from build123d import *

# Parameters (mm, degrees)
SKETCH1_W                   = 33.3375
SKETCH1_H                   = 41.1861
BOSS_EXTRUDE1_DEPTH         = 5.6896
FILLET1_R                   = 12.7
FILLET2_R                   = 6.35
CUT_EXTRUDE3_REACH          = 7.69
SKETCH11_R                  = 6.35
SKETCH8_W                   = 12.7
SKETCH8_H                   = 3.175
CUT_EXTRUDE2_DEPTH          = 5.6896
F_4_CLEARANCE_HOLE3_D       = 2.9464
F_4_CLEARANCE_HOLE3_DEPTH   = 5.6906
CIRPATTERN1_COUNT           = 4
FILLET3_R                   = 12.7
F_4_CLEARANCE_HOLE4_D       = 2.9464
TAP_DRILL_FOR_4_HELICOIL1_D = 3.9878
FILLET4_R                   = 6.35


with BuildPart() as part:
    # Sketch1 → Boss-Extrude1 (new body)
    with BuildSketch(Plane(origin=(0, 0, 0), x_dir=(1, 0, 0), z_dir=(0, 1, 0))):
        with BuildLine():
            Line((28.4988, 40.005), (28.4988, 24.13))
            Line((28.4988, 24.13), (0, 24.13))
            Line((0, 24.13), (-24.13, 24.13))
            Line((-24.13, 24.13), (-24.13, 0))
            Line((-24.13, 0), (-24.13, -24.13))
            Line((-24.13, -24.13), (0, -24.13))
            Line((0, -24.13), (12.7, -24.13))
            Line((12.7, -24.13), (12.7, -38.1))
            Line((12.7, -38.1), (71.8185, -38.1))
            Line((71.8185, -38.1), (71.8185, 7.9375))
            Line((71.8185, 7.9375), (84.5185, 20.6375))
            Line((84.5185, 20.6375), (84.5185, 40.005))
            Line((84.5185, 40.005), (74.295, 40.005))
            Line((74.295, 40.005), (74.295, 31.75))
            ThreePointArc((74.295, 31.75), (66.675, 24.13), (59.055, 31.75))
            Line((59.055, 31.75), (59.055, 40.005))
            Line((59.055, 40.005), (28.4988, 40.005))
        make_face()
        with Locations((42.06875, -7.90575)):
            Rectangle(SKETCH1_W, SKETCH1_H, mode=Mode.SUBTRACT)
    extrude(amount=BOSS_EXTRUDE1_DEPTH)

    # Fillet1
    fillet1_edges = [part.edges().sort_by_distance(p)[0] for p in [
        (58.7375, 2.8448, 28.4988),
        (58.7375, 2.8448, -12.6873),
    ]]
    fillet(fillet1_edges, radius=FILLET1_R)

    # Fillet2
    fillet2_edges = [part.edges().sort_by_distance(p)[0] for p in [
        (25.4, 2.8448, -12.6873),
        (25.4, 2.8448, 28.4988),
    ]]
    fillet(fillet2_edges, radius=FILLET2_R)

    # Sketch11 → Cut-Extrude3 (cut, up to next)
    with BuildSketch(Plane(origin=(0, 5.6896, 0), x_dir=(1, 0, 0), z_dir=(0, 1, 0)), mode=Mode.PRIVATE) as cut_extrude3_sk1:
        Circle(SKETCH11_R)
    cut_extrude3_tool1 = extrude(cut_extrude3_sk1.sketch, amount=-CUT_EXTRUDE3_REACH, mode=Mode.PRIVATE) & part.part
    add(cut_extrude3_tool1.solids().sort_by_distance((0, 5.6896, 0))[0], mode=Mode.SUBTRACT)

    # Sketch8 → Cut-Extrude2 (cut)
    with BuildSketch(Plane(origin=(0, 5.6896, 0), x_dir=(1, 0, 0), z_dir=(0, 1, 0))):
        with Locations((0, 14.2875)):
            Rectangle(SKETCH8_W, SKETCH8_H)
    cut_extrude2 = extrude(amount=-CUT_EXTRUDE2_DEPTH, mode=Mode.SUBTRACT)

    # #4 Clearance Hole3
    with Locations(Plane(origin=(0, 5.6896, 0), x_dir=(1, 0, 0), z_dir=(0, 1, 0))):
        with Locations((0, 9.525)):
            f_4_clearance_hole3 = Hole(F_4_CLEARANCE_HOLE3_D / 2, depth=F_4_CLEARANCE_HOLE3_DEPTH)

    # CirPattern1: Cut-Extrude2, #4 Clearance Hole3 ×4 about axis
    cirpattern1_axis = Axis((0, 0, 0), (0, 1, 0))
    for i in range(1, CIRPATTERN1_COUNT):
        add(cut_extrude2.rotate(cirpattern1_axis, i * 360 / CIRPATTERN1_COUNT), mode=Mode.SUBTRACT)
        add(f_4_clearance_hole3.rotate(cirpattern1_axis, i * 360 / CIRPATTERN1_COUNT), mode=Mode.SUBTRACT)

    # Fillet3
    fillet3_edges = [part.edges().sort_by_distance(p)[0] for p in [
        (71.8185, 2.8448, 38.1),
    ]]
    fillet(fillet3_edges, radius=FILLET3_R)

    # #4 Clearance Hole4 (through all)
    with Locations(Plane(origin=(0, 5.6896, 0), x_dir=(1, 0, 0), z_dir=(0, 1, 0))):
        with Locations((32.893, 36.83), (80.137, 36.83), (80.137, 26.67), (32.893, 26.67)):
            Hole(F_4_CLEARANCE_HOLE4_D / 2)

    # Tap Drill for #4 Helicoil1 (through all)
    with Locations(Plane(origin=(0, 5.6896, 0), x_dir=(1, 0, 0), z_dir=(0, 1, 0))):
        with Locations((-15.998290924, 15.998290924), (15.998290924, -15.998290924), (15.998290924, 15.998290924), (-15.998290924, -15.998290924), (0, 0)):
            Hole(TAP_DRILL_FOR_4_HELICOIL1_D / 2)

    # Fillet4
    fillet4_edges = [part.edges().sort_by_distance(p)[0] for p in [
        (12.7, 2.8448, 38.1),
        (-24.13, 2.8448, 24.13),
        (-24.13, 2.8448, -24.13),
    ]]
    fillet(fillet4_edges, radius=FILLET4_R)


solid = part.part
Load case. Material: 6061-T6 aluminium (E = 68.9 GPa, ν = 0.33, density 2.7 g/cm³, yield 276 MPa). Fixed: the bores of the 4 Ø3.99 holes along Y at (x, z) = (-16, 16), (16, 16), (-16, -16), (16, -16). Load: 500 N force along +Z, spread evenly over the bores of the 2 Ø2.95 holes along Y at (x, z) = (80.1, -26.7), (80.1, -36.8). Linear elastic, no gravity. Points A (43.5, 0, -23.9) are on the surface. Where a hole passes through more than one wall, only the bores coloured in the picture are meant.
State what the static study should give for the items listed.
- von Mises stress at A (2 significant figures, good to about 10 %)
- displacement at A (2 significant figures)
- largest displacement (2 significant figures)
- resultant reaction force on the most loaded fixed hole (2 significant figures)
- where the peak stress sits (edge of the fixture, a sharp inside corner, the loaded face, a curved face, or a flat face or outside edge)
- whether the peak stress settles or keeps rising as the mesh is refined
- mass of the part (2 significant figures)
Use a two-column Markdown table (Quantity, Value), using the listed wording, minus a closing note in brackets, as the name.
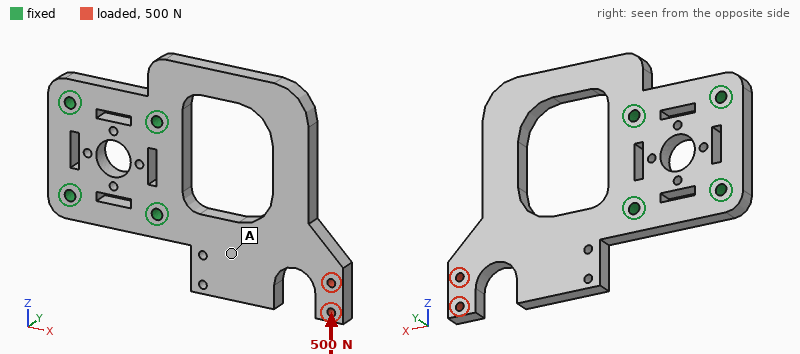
| Quantity | Value |
|---|---|
| von Mises stress at A | 6.6 MPa |
| displacement at A | 0.036 mm |
| largest displacement | 0.12 mm |
| resultant reaction force on the most loaded fixed hole | 640 N |
| where the peak stress sits | edge of the fixture |
| whether the peak stress settles or keeps rising as the mesh is refined | keeps rising |
| mass of the part | 69 g |
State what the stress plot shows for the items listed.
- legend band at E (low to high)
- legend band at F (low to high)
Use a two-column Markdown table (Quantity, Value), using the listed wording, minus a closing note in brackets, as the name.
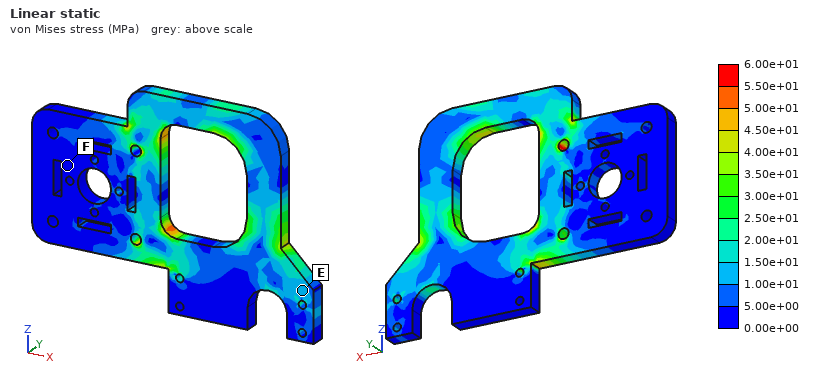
| Quantity | Value |
|---|---|
| legend band at E | 1.00e+01 to 1.50e+01 MPa |
| legend band at F | 0.00e+00 to 5.00e+00 MPa |
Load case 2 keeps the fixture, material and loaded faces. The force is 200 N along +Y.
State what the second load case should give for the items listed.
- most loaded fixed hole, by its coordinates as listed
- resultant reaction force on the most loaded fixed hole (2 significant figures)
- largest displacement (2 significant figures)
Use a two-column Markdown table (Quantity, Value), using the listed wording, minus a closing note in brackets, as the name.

| Quantity | Value |
|---|---|
| most loaded fixed hole, by its coordinates as listed | (16, -16) |
| resultant reaction force on the most loaded fixed hole | 310 N |
| largest displacement | 1.0 mm |
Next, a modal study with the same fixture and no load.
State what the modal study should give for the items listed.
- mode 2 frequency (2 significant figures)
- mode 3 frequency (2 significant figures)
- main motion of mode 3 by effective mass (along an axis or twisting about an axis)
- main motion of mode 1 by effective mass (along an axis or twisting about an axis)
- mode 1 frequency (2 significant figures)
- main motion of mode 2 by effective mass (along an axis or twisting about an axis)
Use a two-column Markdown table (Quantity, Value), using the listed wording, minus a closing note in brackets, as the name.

| Quantity | Value |
|---|---|
| mode 2 frequency | 1700 Hz |
| mode 3 frequency | 2800 Hz |
| main motion of mode 3 by effective mass | along Z |
| main motion of mode 1 by effective mass | along Y |
| mode 1 frequency | 810 Hz |
| main motion of mode 2 by effective mass | twisting about X |
